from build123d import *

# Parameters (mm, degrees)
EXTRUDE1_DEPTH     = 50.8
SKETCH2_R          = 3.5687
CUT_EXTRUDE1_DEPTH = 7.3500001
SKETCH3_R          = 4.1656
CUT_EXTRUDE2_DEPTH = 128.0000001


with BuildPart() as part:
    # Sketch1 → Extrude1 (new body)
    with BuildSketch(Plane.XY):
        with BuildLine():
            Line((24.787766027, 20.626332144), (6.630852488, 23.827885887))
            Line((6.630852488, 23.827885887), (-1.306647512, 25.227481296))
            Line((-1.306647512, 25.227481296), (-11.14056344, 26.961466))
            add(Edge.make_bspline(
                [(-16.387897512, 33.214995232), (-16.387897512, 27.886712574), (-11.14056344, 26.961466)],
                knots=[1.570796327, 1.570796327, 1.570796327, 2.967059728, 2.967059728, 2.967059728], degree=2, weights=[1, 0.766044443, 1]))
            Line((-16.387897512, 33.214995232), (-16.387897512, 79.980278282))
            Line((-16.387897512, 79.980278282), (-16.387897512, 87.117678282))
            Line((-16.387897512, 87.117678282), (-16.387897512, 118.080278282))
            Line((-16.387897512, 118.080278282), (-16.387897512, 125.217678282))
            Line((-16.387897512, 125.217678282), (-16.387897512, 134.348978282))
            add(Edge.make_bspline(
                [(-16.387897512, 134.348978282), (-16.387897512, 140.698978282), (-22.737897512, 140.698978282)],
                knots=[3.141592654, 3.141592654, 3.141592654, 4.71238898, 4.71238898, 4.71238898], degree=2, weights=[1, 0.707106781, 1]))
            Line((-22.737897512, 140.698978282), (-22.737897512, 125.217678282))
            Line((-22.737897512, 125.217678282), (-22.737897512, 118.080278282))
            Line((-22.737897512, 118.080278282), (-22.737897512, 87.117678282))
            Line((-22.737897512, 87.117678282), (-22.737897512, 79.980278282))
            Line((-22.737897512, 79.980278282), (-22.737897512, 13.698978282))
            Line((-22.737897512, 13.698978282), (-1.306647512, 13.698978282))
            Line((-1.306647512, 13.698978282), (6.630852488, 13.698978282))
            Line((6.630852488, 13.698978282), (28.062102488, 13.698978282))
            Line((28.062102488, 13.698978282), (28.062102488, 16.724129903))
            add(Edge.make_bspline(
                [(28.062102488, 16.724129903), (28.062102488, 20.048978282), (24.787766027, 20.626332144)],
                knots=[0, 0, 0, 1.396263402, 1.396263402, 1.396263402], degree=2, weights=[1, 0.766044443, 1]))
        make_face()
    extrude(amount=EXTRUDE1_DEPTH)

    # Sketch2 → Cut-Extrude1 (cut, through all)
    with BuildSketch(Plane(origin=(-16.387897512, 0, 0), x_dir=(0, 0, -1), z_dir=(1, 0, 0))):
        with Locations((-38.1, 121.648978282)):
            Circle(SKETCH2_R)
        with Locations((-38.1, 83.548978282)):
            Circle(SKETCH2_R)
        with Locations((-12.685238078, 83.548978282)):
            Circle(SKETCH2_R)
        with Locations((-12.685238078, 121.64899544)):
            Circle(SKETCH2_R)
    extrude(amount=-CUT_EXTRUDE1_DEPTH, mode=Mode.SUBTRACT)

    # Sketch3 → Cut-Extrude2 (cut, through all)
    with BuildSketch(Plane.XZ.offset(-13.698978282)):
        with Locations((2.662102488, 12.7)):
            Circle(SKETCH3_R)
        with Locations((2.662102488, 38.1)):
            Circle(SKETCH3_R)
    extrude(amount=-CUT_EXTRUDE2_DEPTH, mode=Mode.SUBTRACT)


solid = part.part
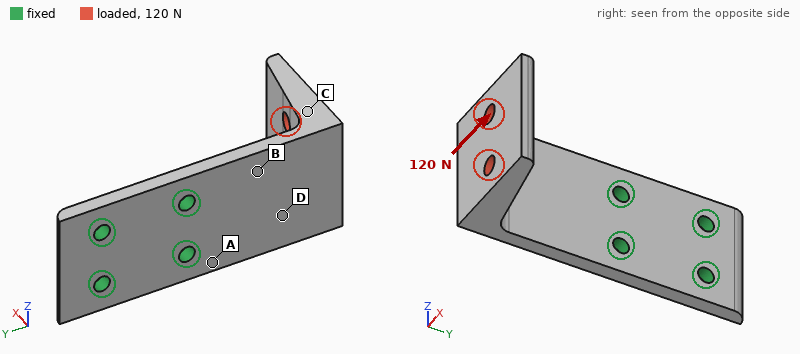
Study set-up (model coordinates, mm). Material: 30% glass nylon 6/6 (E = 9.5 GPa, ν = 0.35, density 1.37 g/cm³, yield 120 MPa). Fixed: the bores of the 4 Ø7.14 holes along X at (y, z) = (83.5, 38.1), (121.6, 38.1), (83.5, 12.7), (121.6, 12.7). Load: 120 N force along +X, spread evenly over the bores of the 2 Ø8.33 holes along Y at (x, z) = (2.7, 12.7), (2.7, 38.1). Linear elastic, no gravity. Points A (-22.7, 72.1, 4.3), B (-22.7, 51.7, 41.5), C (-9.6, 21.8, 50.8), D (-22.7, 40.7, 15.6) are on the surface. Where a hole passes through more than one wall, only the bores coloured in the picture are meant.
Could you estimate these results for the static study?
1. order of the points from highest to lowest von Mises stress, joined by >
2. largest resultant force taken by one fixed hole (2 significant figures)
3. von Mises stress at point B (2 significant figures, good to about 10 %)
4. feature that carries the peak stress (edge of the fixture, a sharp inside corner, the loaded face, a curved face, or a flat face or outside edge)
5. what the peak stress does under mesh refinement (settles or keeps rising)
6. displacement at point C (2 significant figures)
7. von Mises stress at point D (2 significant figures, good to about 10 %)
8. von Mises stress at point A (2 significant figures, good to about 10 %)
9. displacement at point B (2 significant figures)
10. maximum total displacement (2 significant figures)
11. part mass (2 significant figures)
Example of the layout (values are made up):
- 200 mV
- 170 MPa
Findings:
- A > B > D > C
- 70 N
- 11 MPa
- edge of the fixture
- keeps rising
- 0.90 mm
- 7.1 MPa
- 17 MPa
- 0.28 mm
- 1.5 mm
- 85 g
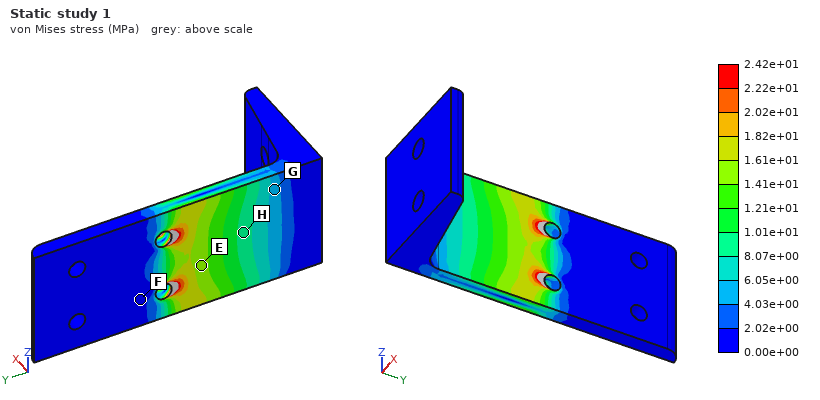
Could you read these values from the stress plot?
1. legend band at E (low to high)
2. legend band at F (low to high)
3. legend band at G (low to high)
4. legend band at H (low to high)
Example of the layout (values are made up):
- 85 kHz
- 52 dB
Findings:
- 1.41e+01 to 1.61e+01 MPa
- 0.00e+00 to 2.02e+00 MPa
- 4.03e+00 to 6.05e+00 MPa
- 8.07e+00 to 1.01e+01 MPa
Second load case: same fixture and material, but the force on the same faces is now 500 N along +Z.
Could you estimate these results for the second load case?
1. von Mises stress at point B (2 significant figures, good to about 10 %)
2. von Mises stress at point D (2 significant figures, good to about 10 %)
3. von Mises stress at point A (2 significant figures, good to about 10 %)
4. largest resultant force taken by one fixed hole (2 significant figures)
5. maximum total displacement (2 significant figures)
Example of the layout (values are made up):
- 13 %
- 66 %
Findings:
- 21 MPa
- 17 MPa
- 25 MPa
- 970 N
- 1.6 mm
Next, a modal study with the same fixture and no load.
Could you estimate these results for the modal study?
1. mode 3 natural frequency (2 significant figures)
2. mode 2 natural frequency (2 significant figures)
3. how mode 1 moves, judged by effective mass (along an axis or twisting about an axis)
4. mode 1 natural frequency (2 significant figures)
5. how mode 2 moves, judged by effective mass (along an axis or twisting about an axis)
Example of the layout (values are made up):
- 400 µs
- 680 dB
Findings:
- 1200 Hz
- 580 Hz
- along X
- 250 Hz
- along Z
